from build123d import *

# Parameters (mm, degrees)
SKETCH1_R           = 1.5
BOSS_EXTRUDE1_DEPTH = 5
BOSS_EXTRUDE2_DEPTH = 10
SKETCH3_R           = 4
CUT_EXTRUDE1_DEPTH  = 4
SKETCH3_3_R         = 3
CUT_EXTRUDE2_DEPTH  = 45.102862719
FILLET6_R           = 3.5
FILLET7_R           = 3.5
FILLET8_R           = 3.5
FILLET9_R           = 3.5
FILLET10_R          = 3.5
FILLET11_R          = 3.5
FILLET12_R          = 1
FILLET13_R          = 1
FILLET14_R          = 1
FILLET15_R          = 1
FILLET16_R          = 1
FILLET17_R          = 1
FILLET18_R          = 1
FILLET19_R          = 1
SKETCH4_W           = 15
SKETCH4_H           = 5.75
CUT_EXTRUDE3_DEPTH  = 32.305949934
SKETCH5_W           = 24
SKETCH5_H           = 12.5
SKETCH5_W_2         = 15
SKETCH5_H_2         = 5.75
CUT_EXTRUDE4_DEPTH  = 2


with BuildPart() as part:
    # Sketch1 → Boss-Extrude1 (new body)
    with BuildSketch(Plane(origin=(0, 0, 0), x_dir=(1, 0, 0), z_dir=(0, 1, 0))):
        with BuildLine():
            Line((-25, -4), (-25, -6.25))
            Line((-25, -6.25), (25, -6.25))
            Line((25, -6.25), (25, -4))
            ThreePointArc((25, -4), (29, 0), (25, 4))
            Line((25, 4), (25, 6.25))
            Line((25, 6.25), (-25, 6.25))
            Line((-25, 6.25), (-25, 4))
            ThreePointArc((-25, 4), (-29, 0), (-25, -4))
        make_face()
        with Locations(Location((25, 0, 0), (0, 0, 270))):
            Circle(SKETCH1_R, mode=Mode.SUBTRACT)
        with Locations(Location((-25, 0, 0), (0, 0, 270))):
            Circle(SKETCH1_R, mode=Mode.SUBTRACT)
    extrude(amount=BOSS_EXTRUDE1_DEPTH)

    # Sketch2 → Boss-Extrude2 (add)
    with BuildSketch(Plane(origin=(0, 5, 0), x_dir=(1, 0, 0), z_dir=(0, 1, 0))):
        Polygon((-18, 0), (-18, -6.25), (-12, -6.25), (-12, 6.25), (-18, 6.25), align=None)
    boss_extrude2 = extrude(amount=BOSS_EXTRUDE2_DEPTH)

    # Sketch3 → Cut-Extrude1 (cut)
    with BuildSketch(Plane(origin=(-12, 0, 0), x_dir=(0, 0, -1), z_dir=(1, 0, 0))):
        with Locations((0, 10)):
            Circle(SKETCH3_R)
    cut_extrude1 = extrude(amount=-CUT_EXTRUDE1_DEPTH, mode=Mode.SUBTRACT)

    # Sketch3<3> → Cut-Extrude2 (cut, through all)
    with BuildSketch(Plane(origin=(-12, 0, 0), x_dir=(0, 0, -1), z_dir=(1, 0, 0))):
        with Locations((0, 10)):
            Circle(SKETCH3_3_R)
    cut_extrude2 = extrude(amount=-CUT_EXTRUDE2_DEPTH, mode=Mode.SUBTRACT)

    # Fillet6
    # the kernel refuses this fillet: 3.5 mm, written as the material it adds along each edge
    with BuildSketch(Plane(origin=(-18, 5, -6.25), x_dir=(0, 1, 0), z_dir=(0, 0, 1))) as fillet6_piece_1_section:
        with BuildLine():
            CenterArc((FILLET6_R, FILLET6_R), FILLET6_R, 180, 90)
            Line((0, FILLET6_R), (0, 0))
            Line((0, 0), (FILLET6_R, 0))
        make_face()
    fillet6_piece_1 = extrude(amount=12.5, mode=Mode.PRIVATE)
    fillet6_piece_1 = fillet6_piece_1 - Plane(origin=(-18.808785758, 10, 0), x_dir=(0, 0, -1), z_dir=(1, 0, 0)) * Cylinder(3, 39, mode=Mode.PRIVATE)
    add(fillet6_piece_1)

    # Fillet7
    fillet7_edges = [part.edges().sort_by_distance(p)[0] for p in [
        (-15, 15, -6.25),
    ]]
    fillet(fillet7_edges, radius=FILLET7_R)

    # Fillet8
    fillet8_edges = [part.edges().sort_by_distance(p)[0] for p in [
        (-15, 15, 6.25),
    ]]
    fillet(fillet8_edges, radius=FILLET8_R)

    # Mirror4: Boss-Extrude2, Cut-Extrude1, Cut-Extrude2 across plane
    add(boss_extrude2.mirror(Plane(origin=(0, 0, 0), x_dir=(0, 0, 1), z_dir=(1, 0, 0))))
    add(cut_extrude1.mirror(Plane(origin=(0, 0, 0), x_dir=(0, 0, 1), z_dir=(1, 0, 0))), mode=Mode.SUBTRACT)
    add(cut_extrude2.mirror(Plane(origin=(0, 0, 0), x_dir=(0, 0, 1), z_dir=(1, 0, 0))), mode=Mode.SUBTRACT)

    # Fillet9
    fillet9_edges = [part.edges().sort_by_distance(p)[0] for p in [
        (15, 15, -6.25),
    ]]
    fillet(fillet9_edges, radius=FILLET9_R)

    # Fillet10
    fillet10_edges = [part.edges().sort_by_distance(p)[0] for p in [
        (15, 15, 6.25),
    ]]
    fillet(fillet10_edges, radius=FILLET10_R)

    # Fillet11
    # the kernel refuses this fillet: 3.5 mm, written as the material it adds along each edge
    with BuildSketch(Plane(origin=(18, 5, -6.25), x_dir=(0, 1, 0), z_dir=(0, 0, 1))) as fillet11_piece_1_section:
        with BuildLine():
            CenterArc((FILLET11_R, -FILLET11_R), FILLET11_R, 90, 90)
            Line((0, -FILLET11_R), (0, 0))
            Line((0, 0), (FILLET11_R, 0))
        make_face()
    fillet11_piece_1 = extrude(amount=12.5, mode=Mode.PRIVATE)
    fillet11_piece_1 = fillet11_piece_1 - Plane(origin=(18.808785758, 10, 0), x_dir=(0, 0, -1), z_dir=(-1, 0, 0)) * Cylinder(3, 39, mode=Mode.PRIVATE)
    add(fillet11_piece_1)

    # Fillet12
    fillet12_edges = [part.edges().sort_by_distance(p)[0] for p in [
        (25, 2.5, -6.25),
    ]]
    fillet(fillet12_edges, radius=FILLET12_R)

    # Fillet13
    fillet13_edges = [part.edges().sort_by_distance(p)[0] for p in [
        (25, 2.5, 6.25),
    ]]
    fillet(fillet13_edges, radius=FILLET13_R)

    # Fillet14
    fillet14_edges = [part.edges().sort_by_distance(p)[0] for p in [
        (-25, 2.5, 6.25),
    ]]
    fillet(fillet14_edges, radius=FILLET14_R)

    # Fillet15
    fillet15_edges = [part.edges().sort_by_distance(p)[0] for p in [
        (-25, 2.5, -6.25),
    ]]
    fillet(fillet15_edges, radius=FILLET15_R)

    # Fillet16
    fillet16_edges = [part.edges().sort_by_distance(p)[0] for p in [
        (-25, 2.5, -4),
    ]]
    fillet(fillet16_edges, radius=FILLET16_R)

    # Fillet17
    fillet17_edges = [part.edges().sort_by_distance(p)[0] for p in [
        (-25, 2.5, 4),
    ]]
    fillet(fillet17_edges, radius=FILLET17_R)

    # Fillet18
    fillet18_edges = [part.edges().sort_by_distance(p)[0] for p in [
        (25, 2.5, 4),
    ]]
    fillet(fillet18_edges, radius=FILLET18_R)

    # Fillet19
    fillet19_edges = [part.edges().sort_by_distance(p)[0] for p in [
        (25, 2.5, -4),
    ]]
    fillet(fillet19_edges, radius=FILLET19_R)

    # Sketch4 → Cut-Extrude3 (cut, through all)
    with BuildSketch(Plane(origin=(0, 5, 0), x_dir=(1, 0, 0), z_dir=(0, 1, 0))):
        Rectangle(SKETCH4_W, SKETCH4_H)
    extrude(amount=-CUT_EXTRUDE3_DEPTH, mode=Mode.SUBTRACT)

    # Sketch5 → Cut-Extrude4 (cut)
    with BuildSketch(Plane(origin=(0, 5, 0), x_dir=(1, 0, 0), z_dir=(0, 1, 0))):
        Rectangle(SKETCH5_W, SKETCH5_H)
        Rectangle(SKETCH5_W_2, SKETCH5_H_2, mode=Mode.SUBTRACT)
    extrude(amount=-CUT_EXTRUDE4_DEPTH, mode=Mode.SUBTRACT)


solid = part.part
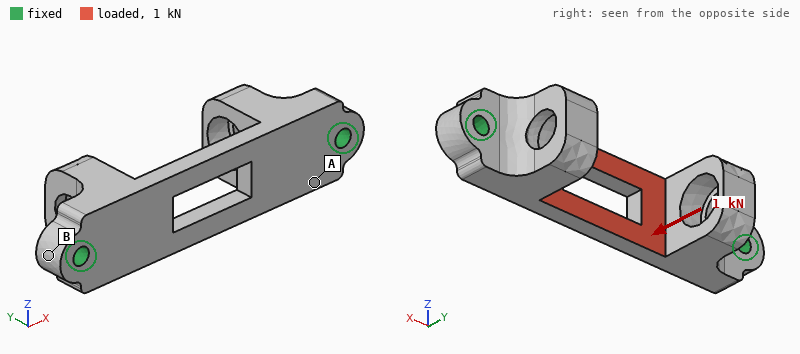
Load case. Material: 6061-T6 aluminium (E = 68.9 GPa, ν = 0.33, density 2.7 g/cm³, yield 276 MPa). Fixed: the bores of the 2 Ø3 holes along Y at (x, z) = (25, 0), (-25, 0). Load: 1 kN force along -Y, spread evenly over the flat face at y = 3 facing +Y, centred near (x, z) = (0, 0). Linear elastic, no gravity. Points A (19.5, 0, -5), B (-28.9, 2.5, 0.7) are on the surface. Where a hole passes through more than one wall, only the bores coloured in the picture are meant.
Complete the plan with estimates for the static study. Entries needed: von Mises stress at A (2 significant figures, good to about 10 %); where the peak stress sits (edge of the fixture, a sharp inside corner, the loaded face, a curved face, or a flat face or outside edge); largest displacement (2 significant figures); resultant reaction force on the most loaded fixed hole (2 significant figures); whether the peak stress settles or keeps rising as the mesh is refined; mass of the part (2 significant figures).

56 MPa
edge of the fixture
0.12 mm
700 N
keeps rising
9.3 g
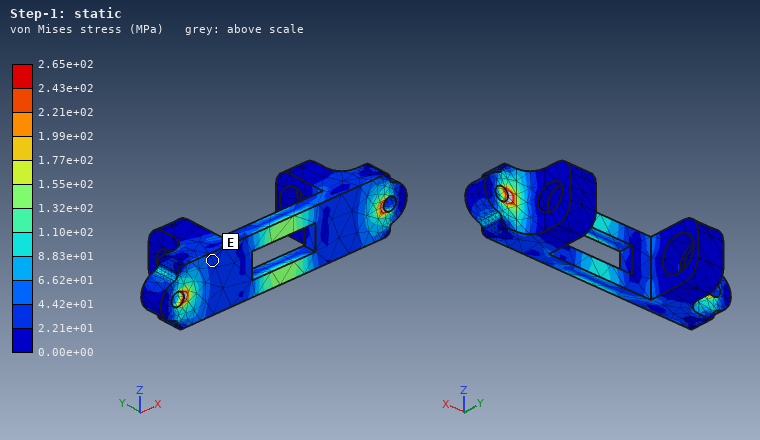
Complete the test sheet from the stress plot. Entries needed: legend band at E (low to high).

2.21e+01 to 4.42e+01 MPa
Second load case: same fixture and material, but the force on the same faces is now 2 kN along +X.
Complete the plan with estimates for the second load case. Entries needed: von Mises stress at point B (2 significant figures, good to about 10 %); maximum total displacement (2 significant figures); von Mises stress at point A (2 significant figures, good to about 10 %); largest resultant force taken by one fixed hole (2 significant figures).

7.5 MPa
12 µm
25 MPa
1.0 kN
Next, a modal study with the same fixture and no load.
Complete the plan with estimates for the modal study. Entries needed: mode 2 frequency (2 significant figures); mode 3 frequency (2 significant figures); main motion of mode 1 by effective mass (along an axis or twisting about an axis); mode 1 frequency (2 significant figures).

13 kHz
14 kHz
along Y
9100 Hz
